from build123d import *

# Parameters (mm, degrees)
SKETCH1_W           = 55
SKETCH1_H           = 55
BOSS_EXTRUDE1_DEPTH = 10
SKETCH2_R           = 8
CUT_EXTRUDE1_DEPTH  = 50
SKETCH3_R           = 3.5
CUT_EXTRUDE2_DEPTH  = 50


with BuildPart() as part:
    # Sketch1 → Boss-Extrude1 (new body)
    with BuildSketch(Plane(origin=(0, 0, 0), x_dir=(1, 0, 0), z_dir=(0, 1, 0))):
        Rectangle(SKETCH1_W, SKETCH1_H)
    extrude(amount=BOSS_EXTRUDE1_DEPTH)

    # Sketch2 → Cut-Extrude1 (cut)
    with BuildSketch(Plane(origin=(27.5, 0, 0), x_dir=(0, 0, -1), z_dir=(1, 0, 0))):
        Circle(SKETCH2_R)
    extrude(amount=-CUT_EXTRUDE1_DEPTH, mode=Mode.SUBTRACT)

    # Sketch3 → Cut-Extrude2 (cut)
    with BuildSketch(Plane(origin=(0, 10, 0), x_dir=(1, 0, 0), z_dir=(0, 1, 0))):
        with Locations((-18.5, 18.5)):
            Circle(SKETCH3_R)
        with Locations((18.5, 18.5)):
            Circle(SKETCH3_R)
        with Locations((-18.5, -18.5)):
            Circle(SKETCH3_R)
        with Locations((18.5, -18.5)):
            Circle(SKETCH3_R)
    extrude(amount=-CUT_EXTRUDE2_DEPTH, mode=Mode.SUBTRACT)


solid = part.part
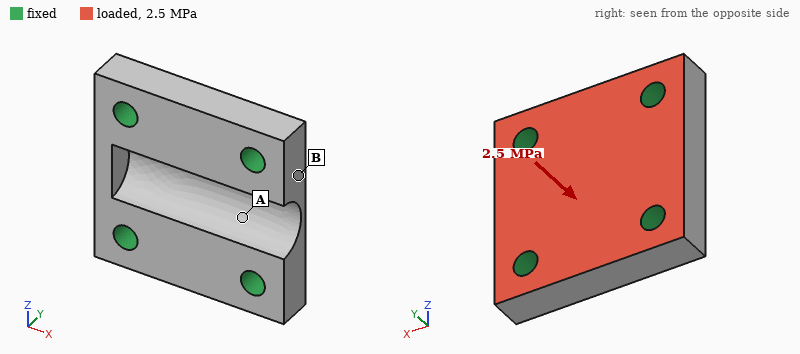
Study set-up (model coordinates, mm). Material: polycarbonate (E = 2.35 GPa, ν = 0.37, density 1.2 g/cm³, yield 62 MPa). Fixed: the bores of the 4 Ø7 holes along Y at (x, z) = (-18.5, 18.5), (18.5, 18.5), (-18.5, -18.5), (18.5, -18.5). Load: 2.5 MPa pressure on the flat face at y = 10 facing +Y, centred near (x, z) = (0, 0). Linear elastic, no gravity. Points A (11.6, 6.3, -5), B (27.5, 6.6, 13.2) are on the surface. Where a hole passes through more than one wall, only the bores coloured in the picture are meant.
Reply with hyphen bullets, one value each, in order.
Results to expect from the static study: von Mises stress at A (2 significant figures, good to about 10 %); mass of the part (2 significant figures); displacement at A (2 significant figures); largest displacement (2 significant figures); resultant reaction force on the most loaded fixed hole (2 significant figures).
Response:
- 13 MPa
- 28 g
- 0.18 mm
- 0.31 mm
- 1.9 kN
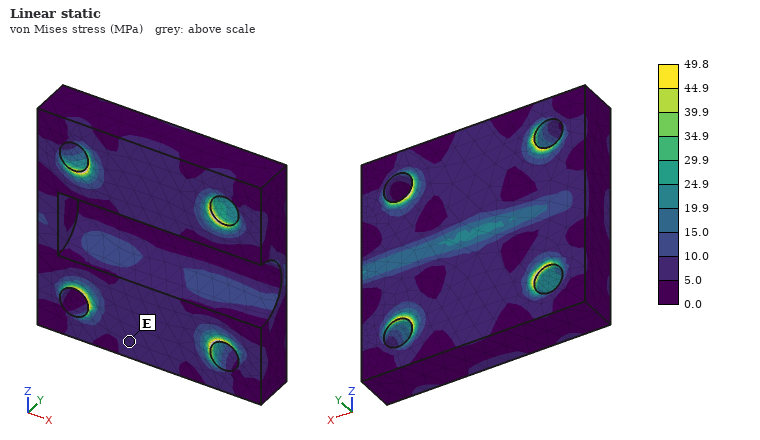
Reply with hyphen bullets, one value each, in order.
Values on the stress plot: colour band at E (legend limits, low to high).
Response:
- 5.0 to 10.0 MPa
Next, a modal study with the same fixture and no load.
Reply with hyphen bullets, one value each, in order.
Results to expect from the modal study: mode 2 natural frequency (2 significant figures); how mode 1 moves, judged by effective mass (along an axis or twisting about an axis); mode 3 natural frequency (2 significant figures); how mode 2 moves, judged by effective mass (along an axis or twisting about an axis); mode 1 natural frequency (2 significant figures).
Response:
- 8300 Hz
- along Y
- 9000 Hz
- twisting about X
- 7200 Hz
